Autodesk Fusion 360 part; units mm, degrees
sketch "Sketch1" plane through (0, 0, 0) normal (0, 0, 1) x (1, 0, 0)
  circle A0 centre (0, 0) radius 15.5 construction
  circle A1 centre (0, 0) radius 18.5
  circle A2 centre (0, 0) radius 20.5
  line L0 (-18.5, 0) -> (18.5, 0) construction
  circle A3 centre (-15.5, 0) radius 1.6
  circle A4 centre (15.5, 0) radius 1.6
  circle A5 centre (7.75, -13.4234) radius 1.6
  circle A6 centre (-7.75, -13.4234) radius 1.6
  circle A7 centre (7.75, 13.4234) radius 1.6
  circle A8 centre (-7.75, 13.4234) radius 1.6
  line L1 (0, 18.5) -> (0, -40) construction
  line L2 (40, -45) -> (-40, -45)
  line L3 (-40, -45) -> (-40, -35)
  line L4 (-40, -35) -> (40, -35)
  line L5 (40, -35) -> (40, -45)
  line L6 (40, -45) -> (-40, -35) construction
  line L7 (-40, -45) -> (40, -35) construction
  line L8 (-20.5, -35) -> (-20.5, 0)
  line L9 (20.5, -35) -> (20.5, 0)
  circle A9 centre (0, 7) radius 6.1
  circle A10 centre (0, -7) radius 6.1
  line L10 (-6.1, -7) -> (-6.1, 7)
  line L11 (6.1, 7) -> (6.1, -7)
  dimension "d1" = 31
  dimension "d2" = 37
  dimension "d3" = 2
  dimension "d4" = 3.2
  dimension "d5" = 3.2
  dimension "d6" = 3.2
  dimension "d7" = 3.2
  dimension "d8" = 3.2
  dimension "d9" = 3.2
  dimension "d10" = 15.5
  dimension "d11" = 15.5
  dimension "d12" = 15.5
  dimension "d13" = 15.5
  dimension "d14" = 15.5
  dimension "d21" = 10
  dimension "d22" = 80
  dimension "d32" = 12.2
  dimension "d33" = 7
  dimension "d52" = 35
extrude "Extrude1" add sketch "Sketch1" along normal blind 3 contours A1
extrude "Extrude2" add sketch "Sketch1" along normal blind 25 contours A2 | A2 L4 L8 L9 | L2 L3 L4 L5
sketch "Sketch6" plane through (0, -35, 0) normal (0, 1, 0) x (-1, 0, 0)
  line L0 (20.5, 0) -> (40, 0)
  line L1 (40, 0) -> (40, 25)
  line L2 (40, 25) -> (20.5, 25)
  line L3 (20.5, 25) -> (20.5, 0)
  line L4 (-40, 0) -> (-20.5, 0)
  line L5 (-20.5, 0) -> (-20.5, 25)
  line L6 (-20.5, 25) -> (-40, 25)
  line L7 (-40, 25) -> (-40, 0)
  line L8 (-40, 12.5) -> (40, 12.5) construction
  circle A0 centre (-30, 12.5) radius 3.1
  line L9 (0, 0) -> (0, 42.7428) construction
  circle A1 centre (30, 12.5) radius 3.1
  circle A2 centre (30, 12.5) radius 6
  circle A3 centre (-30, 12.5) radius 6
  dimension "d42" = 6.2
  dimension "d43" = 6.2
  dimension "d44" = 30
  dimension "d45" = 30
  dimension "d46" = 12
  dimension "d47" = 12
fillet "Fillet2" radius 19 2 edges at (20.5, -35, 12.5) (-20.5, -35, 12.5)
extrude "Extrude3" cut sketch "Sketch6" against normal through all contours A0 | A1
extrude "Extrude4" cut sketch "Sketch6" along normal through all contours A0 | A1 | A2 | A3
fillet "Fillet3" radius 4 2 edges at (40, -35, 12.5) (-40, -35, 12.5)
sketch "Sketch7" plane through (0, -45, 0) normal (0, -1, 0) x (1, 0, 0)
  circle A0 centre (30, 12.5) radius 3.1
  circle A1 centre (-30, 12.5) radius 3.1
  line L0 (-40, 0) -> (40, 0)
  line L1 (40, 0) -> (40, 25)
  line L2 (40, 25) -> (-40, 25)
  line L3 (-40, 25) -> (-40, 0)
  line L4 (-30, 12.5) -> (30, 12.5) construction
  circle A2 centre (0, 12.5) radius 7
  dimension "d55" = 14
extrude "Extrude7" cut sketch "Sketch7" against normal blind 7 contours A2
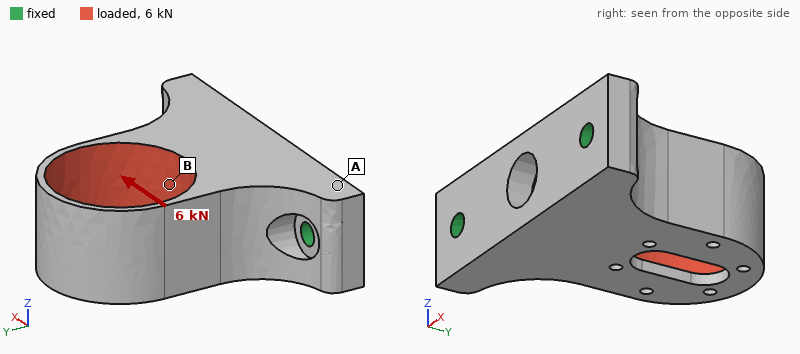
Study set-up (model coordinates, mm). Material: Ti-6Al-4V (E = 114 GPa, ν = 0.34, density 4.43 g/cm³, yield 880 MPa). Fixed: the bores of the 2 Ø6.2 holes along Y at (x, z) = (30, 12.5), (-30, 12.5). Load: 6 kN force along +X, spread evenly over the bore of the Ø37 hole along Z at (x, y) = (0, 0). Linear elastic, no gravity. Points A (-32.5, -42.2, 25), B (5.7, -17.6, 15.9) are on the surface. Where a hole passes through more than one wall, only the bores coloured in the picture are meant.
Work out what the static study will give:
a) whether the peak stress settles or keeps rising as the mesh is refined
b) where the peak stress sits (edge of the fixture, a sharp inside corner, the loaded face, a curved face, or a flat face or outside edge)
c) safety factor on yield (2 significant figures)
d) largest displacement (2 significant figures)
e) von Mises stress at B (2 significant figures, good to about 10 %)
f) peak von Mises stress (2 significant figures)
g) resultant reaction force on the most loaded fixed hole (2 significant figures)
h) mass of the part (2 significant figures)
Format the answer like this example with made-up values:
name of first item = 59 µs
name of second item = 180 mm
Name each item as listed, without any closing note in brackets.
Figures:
whether the peak stress settles or keeps rising as the mesh is refined = settles
where the peak stress sits = a curved face
safety factor on yield = 3.3
largest displacement = 0.22 mm
von Mises stress at B = 40 MPa
peak von Mises stress = 260 MPa
resultant reaction force on the most loaded fixed hole = 5.2 kN
mass of the part = 220 g
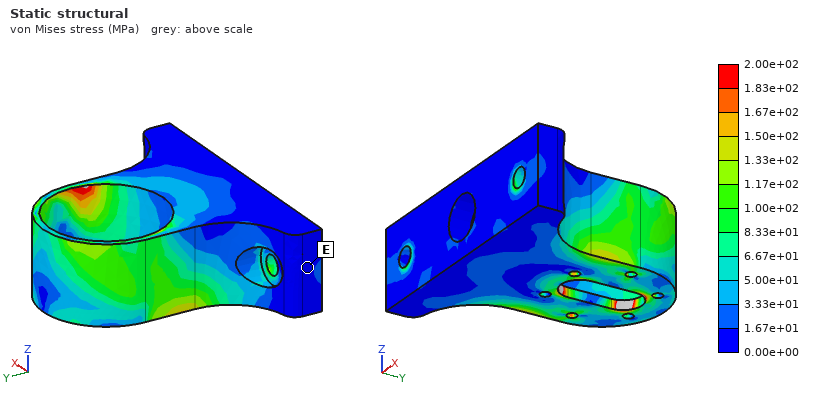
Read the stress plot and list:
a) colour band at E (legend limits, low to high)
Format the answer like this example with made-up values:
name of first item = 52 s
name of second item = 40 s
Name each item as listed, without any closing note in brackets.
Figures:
colour band at E = 0.00e+00 to 1.67e+01 MPa
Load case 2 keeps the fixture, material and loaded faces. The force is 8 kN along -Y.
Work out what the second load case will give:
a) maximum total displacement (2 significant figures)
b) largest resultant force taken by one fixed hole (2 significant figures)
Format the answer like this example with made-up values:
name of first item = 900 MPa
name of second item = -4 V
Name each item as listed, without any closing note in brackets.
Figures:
maximum total displacement = 0.17 mm
largest resultant force taken by one fixed hole = 4.4 kN
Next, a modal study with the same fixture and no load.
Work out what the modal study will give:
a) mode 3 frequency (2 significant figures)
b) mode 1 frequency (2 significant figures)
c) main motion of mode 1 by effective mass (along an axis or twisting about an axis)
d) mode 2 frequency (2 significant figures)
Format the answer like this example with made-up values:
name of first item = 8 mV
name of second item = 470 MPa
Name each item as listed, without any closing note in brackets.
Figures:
mode 3 frequency = 7800 Hz
mode 1 frequency = 3900 Hz
main motion of mode 1 by effective mass = along Z
mode 2 frequency = 5800 Hz
